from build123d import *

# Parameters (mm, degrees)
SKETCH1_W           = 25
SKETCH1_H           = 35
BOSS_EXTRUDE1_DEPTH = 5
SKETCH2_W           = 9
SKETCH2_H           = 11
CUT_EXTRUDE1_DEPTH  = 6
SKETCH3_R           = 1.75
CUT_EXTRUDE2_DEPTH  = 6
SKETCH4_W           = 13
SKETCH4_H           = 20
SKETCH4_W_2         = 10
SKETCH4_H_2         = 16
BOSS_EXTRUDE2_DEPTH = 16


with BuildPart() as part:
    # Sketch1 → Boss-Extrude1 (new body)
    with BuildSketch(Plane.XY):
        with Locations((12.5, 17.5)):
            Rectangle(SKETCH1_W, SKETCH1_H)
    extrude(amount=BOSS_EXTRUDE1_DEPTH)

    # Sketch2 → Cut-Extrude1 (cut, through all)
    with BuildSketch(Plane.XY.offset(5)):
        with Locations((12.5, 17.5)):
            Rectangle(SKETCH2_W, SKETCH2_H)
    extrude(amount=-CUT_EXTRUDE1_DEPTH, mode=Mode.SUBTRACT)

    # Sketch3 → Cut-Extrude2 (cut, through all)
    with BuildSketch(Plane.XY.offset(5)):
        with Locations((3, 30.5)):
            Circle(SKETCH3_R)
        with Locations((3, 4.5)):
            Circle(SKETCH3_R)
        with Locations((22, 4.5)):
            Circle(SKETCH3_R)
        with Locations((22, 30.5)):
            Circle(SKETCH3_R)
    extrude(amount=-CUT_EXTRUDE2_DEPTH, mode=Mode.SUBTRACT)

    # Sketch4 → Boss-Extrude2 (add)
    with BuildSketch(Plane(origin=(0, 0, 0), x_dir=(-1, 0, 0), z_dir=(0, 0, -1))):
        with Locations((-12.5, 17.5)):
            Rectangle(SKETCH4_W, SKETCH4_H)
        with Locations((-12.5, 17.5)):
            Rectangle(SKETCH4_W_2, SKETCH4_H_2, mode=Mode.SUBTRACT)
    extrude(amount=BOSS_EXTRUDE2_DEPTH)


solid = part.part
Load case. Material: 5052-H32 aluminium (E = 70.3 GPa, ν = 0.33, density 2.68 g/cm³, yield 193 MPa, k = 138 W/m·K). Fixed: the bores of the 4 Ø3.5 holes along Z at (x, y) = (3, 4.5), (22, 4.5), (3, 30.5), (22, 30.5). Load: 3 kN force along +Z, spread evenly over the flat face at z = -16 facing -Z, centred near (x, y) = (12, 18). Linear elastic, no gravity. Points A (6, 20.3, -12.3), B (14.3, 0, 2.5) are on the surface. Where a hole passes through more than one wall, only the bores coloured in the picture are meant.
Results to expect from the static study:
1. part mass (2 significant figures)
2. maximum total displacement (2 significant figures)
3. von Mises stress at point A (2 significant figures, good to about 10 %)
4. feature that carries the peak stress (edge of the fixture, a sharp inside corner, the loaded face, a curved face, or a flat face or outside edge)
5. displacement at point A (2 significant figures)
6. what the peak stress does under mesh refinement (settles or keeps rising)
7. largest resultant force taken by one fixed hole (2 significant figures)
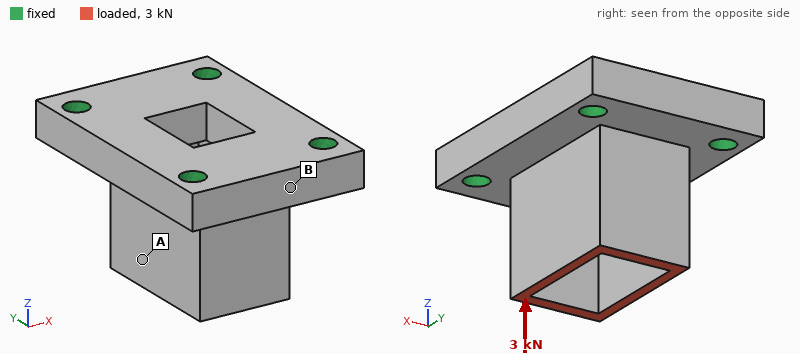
14 g
15 µm
27 MPa
edge of the fixture
14 µm
keeps rising
780 N
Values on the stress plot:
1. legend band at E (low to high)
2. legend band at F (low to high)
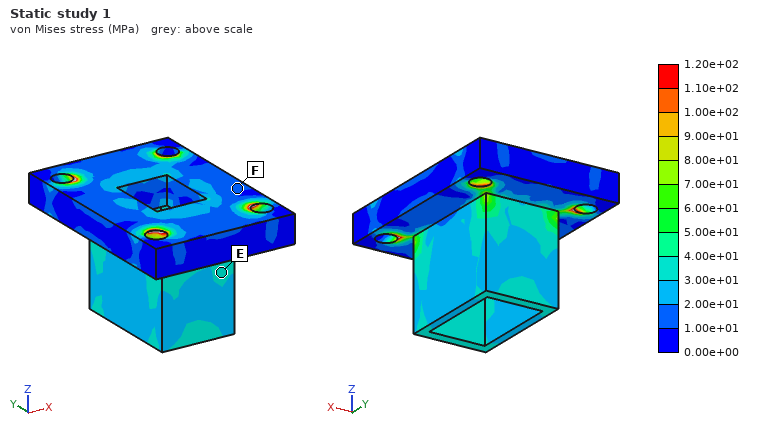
3.00e+01 to 4.00e+01 MPa
1.00e+01 to 2.00e+01 MPa
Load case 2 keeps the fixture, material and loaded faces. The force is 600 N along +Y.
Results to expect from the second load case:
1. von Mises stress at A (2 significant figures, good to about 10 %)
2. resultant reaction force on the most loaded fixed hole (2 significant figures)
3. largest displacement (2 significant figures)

26 MPa
300 N
24 µm
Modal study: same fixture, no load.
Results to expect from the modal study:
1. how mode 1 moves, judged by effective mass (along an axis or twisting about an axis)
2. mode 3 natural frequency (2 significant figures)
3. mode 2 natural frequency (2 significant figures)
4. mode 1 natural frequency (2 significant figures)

along X
23 kHz
21 kHz
18 kHz
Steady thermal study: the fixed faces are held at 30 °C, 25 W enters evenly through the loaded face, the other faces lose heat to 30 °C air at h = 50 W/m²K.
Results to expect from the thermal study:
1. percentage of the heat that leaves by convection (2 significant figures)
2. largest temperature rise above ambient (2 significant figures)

8.6 %
34 K
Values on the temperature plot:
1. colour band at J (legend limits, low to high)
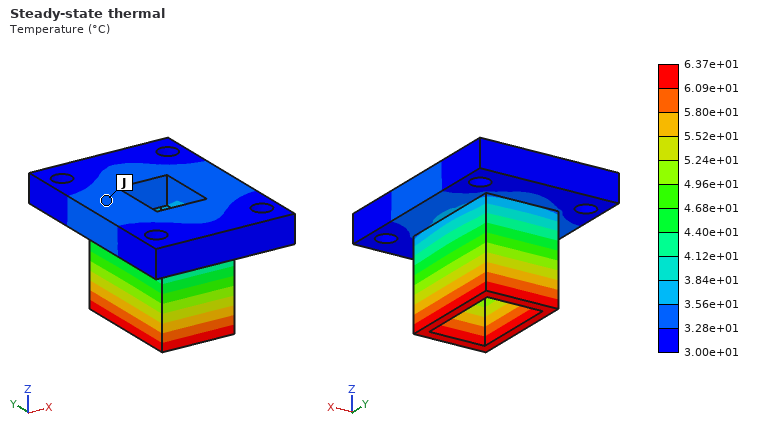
3.28e+01 to 3.56e+01 °C
